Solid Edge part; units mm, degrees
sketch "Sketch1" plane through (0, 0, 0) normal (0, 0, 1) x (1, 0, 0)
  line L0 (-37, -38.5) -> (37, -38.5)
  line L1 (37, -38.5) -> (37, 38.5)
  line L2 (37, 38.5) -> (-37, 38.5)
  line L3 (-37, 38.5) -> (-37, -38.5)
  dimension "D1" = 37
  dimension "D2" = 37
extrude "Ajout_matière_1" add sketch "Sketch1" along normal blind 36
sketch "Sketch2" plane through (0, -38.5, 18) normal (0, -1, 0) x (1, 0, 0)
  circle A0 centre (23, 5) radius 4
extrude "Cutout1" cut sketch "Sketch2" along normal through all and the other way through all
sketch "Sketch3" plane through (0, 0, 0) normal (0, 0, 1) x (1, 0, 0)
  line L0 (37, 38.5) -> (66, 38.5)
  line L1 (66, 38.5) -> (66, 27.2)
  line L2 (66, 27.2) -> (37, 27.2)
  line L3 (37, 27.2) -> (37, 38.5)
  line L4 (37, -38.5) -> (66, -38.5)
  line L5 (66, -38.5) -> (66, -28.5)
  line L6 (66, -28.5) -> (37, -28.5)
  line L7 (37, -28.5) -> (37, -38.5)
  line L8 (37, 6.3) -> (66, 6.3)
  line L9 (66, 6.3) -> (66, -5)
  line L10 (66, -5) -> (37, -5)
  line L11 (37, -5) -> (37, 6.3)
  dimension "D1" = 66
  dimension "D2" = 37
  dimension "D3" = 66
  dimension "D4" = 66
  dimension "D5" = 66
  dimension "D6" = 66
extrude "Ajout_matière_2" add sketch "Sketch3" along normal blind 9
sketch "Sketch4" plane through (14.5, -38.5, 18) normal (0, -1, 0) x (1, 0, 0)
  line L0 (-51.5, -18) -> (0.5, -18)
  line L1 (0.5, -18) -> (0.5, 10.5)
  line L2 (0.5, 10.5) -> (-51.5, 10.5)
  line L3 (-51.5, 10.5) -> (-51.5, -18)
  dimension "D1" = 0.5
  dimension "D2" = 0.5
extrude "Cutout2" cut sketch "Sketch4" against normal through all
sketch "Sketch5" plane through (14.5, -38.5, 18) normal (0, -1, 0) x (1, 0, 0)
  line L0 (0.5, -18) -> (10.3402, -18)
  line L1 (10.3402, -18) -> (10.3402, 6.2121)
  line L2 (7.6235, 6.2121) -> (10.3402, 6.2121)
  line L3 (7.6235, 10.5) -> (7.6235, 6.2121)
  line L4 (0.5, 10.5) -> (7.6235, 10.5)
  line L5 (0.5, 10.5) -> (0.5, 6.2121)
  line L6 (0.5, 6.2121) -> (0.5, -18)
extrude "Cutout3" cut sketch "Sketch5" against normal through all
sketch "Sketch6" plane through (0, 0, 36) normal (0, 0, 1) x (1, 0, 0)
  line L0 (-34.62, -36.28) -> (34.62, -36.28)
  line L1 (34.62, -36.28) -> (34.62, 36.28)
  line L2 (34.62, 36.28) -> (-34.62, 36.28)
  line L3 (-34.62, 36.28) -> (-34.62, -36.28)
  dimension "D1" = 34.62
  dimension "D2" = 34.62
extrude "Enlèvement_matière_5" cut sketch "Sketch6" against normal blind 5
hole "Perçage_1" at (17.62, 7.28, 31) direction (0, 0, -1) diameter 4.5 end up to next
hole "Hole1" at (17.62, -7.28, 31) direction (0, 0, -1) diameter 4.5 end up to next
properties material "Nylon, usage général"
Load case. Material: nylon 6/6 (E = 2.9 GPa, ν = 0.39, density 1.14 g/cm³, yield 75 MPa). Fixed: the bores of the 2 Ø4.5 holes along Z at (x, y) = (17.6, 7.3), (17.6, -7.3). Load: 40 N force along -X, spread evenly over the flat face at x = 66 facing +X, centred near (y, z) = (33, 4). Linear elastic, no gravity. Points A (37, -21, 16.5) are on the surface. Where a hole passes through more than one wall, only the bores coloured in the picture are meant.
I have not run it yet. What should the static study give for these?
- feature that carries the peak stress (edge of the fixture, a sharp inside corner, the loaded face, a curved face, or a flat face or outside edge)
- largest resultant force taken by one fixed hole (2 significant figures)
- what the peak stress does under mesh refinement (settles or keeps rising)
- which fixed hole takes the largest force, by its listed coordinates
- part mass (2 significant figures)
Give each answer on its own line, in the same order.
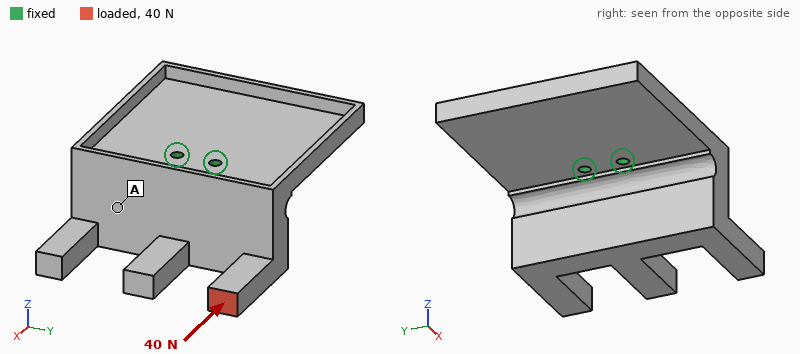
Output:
edge of the fixture
95 N
keeps rising
(17.6, 7.3)
60 g
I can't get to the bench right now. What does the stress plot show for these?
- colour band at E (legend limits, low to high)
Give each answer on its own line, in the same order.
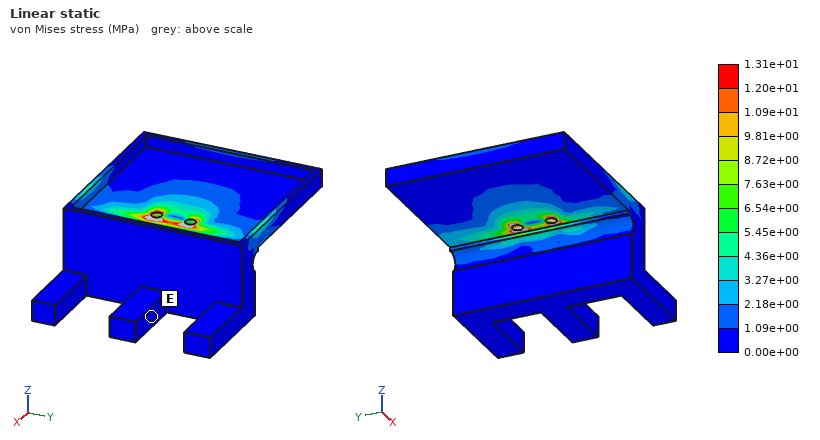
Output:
0.00e+00 to 1.09e+00 MPa
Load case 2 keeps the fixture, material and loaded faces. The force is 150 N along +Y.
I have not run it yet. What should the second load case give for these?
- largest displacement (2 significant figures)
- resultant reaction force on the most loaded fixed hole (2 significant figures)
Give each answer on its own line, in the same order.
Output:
1.5 mm
480 N
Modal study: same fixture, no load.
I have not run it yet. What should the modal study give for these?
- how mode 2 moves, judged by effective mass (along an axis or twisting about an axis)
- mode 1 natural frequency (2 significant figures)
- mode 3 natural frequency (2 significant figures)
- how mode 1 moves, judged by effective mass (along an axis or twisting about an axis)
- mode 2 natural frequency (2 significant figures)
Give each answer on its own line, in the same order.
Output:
along Z
160 Hz
370 Hz
along X
320 Hz
